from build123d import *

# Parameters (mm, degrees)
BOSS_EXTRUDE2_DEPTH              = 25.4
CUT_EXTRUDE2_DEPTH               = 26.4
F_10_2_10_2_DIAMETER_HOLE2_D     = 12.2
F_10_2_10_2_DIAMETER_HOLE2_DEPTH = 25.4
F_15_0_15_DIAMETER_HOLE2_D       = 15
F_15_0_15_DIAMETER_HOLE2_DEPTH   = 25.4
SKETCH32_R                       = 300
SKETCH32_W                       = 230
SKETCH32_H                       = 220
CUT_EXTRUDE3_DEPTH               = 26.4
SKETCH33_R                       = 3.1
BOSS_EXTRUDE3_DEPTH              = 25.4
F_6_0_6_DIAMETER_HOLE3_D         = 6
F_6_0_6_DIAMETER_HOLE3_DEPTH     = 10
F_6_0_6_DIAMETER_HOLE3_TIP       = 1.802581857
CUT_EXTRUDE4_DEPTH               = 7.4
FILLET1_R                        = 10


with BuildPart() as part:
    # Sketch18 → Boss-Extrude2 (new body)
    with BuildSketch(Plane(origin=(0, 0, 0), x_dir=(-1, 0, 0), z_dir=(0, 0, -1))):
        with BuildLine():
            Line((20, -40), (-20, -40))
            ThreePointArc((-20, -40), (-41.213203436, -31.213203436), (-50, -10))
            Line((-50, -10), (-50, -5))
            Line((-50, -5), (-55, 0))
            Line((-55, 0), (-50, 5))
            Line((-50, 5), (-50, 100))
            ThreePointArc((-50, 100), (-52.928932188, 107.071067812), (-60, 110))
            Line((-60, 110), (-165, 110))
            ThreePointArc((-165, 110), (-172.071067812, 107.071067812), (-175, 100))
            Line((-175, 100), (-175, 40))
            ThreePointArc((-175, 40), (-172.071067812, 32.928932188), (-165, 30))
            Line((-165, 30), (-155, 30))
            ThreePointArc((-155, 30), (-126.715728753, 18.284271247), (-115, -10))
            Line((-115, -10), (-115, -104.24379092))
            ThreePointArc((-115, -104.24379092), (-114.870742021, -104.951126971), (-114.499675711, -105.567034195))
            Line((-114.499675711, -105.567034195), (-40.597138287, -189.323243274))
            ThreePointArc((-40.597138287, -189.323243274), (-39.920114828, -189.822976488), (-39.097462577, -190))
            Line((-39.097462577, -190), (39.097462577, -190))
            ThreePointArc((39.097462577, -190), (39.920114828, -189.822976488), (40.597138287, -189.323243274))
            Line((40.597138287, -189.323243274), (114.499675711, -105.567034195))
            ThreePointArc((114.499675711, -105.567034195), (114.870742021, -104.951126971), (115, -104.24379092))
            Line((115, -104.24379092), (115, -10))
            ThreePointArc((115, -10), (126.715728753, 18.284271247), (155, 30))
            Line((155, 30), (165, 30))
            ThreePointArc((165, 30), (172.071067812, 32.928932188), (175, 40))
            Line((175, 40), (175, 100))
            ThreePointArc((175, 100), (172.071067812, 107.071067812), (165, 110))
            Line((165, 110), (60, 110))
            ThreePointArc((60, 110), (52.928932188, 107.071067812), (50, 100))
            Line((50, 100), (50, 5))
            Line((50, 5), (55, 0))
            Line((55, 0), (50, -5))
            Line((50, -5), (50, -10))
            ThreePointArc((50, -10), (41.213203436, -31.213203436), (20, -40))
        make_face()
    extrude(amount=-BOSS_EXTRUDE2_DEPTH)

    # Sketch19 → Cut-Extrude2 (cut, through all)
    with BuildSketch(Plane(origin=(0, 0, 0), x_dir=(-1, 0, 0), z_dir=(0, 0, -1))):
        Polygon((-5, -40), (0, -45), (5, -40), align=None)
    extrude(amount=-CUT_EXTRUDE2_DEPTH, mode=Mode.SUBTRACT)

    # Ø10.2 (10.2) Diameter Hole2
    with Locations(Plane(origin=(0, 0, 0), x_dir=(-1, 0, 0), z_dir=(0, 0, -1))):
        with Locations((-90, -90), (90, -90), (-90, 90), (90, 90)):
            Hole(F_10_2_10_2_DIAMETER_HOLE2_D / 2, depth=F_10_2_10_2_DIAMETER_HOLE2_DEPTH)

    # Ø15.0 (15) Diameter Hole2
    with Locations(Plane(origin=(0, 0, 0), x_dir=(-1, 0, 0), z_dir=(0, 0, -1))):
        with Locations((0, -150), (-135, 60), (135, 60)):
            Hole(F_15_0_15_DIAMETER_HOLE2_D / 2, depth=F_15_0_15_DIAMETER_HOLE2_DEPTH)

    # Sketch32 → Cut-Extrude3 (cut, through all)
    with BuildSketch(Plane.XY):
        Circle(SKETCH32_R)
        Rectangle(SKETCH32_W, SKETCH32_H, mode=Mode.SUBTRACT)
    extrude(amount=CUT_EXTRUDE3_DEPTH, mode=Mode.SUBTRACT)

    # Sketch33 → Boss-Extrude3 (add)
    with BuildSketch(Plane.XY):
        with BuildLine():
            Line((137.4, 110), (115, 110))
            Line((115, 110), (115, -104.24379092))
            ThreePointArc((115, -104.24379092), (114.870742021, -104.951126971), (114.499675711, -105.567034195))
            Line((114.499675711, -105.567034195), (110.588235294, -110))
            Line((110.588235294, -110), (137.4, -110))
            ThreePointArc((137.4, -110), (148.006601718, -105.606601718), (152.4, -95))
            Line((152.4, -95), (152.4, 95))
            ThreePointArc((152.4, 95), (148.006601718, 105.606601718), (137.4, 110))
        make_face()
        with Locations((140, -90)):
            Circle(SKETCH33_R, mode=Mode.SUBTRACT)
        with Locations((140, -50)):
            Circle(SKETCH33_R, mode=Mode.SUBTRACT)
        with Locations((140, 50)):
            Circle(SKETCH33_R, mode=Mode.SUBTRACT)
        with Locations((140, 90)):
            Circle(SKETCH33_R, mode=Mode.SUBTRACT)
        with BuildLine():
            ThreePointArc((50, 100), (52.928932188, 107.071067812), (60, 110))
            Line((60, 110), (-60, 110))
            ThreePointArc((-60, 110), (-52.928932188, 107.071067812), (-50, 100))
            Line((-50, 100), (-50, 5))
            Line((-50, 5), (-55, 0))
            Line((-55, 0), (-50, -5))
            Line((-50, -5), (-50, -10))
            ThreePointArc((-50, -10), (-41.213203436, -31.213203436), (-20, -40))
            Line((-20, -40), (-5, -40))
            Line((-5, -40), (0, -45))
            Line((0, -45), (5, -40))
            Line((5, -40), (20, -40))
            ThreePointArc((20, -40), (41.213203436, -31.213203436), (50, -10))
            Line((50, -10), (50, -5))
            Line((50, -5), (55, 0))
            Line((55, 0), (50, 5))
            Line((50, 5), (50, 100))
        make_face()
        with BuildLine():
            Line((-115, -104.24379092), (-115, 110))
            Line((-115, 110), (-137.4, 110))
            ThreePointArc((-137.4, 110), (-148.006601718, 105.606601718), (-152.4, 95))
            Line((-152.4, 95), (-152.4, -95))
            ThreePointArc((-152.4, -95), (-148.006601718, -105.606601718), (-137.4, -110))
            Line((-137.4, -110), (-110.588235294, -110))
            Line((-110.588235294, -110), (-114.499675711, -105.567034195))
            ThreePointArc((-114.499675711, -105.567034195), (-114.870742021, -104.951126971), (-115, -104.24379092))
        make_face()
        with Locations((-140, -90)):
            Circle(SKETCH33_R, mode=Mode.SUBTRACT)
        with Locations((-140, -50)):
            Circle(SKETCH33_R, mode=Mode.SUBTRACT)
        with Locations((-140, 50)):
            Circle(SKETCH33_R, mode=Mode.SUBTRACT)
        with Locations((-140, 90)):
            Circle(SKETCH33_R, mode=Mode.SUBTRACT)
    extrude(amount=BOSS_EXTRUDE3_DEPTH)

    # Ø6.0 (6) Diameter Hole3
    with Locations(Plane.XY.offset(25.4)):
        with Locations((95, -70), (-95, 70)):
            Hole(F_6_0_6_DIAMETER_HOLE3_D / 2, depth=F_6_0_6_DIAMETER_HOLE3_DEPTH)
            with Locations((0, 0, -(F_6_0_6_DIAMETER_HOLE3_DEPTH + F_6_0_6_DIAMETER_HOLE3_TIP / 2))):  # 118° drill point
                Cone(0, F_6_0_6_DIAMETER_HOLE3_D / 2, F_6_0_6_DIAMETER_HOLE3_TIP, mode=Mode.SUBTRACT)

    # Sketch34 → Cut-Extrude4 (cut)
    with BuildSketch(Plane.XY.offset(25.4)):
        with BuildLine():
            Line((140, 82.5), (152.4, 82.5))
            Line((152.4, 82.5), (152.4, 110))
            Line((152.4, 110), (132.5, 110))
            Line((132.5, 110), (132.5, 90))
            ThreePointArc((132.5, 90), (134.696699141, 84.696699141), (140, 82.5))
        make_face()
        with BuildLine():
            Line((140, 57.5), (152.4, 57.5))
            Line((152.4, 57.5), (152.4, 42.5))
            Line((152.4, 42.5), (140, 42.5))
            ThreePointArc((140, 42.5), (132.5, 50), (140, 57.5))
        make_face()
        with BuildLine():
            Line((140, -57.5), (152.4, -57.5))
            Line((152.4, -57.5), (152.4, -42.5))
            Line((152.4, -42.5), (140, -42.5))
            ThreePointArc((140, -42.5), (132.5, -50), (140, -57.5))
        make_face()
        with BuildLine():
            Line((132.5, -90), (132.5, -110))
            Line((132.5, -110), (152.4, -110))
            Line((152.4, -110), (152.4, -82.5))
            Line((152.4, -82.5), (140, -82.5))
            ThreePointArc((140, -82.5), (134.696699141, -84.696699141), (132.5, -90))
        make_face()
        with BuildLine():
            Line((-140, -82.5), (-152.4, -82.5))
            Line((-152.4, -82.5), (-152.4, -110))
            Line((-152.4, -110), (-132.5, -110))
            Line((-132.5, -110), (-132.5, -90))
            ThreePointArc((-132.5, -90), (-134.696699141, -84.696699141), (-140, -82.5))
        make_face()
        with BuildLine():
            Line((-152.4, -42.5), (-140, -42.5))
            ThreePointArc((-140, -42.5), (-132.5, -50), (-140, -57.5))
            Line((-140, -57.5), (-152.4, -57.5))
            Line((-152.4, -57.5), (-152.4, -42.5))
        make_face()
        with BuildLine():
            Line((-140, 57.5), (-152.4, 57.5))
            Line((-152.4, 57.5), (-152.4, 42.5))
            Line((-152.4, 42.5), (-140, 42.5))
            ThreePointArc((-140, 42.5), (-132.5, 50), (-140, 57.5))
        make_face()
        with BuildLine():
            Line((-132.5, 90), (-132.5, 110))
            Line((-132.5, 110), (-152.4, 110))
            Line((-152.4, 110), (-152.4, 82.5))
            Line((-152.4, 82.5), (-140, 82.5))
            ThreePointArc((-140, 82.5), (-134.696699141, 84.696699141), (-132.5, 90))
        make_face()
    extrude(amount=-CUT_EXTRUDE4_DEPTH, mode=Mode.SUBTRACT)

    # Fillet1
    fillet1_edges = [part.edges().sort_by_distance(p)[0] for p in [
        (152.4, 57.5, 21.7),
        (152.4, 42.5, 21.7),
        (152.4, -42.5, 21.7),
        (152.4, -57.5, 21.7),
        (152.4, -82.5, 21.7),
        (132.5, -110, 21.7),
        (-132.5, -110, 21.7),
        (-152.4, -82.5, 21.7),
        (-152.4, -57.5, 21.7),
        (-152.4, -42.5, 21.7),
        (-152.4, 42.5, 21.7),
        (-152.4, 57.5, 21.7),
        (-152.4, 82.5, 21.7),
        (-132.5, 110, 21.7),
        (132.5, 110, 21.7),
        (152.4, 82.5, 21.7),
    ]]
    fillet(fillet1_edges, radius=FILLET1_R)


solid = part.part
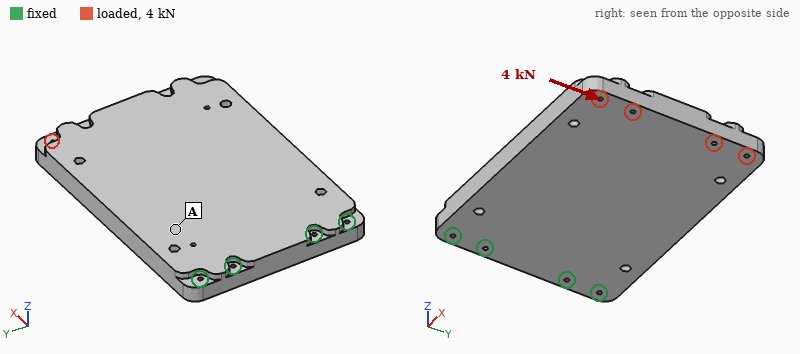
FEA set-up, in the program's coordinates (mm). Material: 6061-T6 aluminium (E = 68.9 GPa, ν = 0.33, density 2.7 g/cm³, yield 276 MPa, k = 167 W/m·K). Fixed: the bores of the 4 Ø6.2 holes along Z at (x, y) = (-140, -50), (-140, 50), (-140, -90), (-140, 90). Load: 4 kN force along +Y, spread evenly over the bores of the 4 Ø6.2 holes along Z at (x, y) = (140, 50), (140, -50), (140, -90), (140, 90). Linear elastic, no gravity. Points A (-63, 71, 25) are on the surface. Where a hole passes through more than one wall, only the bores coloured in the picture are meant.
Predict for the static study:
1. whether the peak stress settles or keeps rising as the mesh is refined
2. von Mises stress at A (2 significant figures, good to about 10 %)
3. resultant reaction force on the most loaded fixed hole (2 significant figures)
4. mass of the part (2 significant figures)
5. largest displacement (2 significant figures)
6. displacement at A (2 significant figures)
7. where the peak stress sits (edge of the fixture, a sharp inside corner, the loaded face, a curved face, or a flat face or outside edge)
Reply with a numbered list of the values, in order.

1. keeps rising
2. 2.4 MPa
3. 5.0 kN
4. 4.5 kg
5. 46 µm
6. 9.8 µm
7. edge of the fixture
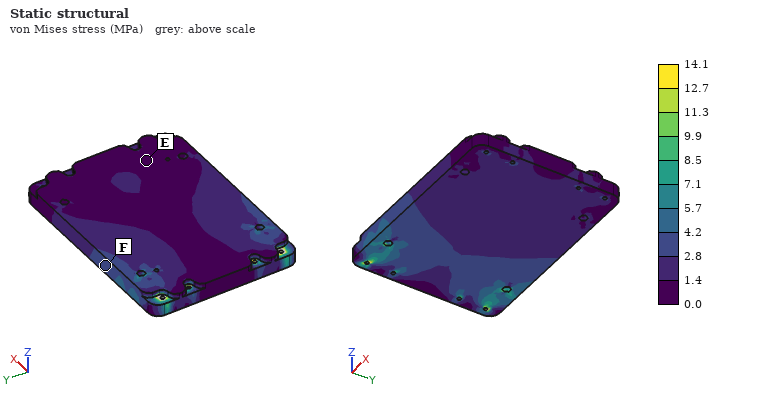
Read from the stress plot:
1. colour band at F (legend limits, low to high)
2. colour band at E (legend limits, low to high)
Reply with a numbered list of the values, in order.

1. 2.8 to 4.2 MPa
2. 0.0 to 1.4 MPa
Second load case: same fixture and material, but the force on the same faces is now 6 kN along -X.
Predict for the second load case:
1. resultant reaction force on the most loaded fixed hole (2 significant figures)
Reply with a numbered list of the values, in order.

1. 1.7 kN
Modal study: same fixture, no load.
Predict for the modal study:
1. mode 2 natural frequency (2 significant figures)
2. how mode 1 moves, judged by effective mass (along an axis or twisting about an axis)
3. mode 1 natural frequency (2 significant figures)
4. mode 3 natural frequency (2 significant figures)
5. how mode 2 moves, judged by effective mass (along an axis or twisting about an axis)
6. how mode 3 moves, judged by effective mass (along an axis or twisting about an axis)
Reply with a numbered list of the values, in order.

1. 680 Hz
2. along Z
3. 190 Hz
4. 1300 Hz
5. twisting about X
6. along Z
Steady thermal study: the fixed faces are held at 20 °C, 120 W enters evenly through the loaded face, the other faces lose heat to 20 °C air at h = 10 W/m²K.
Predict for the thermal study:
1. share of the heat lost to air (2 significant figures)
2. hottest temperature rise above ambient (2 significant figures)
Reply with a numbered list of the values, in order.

1. 23 %
2. 37 K
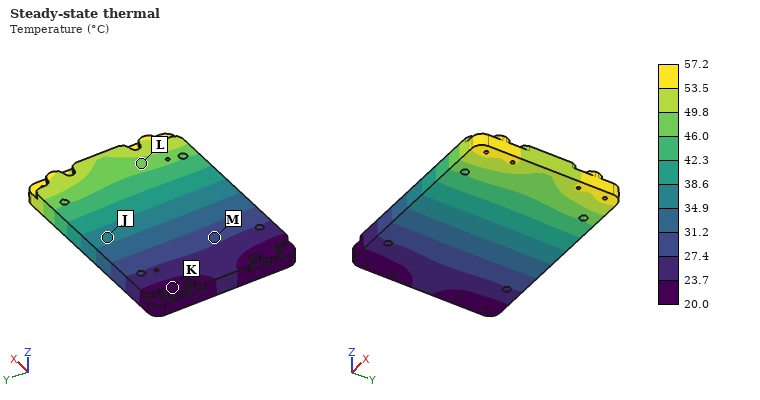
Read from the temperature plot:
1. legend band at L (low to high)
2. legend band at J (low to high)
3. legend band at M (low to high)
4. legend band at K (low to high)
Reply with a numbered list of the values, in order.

1. 46.0 to 49.8 °C
2. 34.9 to 38.6 °C
3. 27.4 to 31.2 °C
4. 20.0 to 23.7 °C
